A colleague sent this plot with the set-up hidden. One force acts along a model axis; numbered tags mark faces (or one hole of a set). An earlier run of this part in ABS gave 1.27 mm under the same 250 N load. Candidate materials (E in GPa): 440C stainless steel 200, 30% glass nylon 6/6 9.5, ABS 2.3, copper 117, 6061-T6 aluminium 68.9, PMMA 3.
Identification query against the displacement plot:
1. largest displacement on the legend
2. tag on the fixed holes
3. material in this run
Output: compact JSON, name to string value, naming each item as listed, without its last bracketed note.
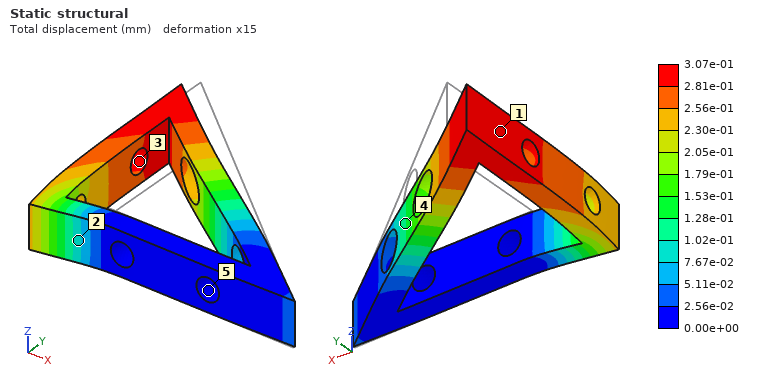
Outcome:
{"largest displacement on the legend": "3.07e-01 mm", "tag on the fixed holes": "5", "material in this run": "30% glass nylon 6/6"}
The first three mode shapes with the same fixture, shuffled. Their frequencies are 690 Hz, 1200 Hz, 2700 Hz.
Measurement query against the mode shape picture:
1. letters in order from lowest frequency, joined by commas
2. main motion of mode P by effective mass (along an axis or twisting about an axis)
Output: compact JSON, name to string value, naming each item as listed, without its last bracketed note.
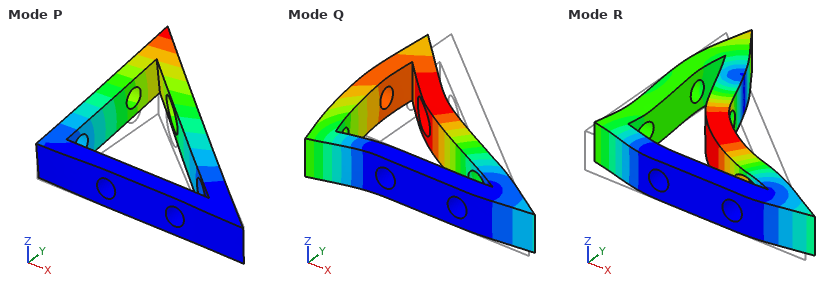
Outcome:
{"letters in order from lowest frequency, joined by commas": "P, Q, R", "main motion of mode P by effective mass": "along Z"}
